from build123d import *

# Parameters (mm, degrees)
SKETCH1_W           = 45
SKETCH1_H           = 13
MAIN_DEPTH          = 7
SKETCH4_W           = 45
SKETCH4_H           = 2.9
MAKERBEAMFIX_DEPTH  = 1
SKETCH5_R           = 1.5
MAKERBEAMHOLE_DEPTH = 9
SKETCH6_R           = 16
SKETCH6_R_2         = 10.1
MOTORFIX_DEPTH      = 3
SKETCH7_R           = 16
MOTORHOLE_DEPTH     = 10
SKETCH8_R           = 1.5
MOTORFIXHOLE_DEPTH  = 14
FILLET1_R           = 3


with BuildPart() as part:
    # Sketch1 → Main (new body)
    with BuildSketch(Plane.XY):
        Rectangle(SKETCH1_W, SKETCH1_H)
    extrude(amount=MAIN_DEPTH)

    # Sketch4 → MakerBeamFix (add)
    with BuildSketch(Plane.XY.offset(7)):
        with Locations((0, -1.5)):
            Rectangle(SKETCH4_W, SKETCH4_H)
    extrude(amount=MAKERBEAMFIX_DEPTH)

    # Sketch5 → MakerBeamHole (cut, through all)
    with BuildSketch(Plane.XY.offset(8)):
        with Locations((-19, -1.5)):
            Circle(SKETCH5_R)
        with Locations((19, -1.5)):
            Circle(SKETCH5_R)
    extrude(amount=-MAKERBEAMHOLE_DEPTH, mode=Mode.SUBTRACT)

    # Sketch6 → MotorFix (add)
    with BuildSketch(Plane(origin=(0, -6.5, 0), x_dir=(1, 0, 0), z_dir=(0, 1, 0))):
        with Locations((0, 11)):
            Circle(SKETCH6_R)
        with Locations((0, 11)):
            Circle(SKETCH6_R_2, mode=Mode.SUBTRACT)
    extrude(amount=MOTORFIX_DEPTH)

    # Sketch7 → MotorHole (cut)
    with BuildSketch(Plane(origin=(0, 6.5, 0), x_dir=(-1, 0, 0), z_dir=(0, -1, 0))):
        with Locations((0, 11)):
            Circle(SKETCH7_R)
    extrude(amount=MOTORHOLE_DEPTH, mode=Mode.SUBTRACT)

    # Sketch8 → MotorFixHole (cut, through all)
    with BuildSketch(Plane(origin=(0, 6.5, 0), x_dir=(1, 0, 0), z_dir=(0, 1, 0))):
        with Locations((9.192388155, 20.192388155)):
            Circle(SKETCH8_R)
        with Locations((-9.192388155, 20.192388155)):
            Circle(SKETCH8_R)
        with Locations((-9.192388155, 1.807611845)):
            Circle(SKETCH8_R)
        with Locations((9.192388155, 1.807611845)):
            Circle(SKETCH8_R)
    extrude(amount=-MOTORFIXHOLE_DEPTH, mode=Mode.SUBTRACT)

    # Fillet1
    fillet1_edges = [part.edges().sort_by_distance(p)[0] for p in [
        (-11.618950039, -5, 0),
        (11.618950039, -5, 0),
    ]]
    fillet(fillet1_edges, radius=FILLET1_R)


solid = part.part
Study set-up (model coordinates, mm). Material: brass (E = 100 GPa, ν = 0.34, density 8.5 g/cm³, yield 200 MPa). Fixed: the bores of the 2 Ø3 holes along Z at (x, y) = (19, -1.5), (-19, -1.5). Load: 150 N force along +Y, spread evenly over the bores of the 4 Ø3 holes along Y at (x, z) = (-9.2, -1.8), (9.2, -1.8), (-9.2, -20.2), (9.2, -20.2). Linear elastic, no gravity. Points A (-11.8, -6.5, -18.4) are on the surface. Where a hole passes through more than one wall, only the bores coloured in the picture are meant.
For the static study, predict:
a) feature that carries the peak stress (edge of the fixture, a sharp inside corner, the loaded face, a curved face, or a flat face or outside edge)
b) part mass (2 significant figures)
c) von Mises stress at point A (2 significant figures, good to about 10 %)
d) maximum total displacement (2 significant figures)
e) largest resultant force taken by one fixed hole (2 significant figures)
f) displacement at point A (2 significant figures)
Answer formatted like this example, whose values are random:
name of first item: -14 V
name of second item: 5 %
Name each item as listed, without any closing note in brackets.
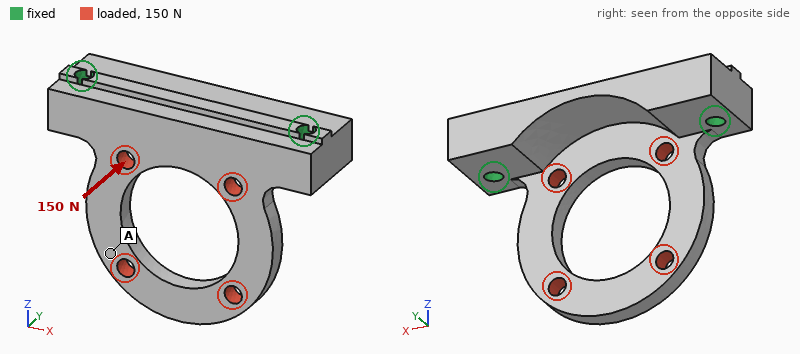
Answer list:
feature that carries the peak stress: the loaded face
part mass: 38 g
von Mises stress at point A: 14 MPa
maximum total displacement: 0.16 mm
largest resultant force taken by one fixed hole: 75 N
displacement at point A: 0.093 mm
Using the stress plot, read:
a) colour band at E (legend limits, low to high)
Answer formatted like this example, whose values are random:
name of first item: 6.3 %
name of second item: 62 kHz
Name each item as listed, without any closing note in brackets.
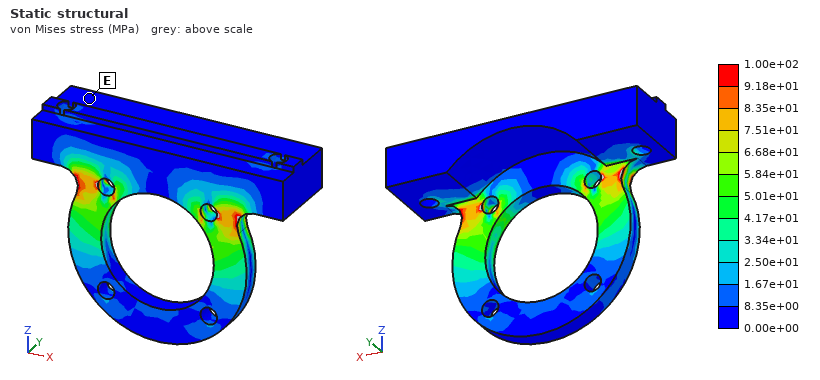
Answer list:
colour band at E: 0.00e+00 to 8.35e+00 MPa
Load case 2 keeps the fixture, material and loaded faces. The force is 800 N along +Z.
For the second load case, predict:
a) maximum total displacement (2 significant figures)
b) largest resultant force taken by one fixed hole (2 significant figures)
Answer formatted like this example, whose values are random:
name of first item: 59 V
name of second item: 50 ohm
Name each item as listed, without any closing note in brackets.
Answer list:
maximum total displacement: 14 µm
largest resultant force taken by one fixed hole: 400 N
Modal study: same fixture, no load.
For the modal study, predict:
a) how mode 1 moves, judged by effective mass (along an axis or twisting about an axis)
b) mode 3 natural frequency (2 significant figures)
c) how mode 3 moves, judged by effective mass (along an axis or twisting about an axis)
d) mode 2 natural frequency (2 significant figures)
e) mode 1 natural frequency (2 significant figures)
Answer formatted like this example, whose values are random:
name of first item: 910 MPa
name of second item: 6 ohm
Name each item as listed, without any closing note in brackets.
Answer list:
how mode 1 moves, judged by effective mass: along Y
mode 3 natural frequency: 7000 Hz
how mode 3 moves, judged by effective mass: along X
mode 2 natural frequency: 4500 Hz
mode 1 natural frequency: 1800 Hz
